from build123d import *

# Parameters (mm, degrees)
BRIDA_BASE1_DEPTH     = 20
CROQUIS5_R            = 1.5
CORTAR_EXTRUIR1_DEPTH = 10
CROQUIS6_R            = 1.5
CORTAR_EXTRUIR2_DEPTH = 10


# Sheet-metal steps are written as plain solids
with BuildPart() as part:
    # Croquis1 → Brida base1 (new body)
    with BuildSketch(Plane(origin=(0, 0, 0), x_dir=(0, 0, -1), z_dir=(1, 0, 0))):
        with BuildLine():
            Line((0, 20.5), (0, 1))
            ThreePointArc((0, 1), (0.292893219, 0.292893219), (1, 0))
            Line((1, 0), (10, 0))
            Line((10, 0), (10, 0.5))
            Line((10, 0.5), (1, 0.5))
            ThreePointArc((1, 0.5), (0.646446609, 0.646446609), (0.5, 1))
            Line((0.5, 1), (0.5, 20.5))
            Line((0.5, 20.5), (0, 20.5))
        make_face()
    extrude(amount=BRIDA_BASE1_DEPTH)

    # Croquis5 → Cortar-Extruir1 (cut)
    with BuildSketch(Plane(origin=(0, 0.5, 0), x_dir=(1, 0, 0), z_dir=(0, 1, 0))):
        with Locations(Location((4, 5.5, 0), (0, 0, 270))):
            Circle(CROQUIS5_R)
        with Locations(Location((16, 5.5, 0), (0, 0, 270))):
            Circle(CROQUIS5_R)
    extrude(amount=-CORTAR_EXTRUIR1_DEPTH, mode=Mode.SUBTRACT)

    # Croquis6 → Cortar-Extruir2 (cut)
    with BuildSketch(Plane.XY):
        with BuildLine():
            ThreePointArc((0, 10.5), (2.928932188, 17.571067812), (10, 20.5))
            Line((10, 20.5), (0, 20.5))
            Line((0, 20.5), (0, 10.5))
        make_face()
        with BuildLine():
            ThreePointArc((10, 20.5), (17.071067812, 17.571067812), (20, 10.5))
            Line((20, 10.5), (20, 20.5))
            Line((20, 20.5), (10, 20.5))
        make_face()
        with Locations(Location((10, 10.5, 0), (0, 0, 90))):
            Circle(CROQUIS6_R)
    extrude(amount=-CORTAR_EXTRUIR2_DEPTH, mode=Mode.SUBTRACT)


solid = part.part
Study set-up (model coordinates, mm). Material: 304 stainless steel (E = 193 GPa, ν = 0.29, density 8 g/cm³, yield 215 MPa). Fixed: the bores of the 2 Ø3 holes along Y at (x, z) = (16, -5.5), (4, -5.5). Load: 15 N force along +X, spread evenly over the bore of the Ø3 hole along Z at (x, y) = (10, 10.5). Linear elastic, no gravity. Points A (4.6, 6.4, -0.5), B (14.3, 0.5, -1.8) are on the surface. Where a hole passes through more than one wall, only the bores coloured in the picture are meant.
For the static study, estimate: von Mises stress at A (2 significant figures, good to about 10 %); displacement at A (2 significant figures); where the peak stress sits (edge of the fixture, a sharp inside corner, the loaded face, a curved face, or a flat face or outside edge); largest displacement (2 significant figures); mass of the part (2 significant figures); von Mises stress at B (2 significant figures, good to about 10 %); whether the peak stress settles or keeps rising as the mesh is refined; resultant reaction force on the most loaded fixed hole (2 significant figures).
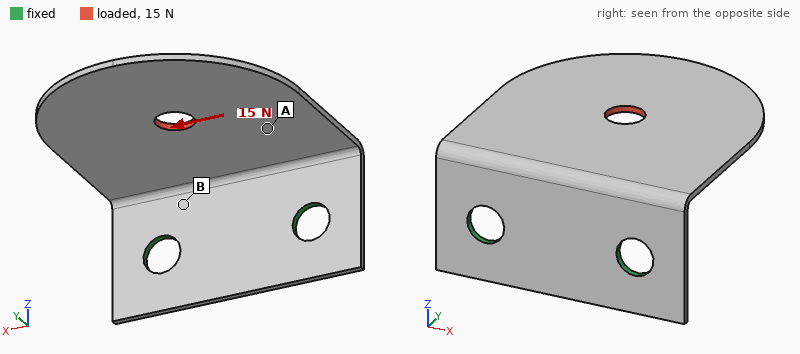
14 MPa
17 µm
edge of the fixture
36 µm
2.1 g
45 MPa
keeps rising
15 N
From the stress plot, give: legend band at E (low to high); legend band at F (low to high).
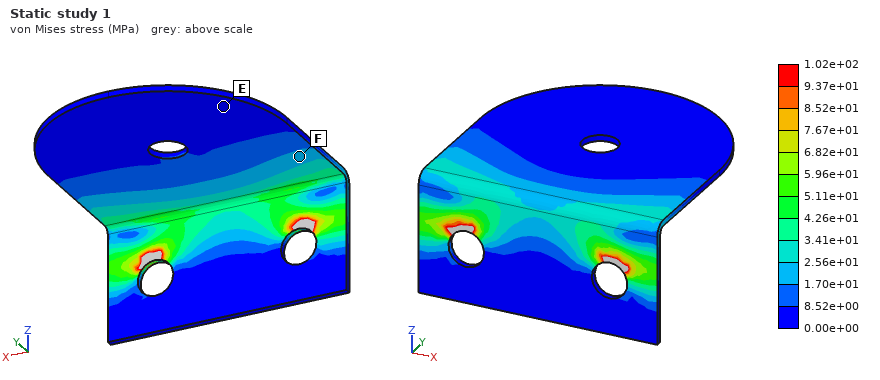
0.00e+00 to 8.52e+00 MPa
1.70e+01 to 2.56e+01 MPa
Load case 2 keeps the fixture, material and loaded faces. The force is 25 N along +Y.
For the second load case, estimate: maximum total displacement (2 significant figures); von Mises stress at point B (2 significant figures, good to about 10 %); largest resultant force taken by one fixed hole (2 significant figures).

0.11 mm
50 MPa
13 N
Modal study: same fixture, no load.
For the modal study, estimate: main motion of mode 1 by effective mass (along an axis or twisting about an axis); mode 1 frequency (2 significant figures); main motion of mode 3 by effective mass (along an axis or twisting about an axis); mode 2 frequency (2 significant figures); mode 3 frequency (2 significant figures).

along Z
880 Hz
along X
2600 Hz
4000 Hz
